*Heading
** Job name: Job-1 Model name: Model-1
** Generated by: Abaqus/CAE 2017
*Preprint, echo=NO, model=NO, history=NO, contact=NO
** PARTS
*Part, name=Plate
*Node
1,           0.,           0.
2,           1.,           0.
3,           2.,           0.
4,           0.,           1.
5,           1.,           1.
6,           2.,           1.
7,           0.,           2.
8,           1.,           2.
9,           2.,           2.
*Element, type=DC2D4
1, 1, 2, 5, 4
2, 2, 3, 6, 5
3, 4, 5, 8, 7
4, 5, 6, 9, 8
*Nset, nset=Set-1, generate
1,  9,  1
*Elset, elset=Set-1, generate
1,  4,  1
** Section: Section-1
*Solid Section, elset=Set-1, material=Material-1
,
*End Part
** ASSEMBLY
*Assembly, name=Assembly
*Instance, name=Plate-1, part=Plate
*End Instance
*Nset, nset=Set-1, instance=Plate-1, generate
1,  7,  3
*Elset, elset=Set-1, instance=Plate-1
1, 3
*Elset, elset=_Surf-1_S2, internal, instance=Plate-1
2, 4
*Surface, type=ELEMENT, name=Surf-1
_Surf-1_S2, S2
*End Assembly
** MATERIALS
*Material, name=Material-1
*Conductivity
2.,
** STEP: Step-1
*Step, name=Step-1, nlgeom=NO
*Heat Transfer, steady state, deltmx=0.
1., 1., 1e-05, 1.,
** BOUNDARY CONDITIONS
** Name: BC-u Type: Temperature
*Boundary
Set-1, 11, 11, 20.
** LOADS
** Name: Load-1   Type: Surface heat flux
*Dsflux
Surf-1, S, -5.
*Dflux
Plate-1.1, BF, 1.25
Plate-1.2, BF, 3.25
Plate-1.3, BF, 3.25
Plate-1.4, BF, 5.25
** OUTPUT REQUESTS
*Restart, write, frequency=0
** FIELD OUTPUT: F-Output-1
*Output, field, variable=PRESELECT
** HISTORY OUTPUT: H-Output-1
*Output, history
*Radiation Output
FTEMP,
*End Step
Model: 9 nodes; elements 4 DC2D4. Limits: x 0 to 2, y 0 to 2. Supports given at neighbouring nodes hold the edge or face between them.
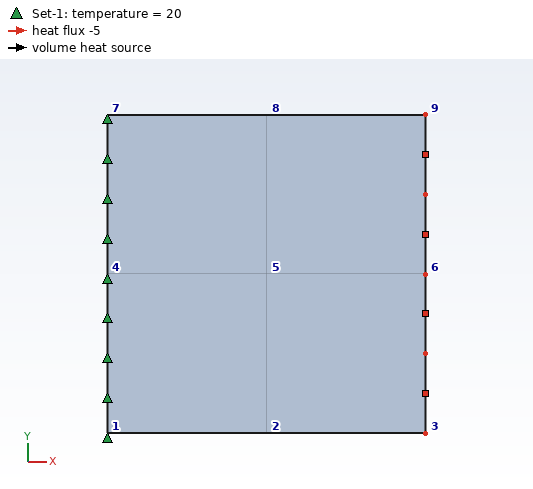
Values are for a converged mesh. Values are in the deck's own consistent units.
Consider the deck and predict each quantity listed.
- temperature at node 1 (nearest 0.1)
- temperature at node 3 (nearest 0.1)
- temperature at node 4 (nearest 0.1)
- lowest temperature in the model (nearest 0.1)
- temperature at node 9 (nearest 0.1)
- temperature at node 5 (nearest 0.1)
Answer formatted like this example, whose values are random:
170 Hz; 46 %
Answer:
20.0; 18.5; 20.0; 18.5; 19.0; 20.2
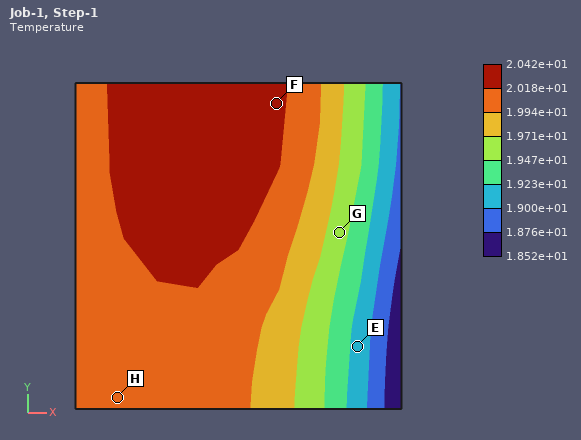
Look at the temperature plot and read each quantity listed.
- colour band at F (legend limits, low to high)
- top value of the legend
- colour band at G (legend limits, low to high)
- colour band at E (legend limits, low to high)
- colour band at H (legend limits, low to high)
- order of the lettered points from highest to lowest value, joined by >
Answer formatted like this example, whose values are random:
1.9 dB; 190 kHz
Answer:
2.018e+01 to 2.042e+01; 2.042e+01; 1.947e+01 to 1.971e+01; 1.900e+01 to 1.923e+01; 1.994e+01 to 2.018e+01; F > H > G > E
